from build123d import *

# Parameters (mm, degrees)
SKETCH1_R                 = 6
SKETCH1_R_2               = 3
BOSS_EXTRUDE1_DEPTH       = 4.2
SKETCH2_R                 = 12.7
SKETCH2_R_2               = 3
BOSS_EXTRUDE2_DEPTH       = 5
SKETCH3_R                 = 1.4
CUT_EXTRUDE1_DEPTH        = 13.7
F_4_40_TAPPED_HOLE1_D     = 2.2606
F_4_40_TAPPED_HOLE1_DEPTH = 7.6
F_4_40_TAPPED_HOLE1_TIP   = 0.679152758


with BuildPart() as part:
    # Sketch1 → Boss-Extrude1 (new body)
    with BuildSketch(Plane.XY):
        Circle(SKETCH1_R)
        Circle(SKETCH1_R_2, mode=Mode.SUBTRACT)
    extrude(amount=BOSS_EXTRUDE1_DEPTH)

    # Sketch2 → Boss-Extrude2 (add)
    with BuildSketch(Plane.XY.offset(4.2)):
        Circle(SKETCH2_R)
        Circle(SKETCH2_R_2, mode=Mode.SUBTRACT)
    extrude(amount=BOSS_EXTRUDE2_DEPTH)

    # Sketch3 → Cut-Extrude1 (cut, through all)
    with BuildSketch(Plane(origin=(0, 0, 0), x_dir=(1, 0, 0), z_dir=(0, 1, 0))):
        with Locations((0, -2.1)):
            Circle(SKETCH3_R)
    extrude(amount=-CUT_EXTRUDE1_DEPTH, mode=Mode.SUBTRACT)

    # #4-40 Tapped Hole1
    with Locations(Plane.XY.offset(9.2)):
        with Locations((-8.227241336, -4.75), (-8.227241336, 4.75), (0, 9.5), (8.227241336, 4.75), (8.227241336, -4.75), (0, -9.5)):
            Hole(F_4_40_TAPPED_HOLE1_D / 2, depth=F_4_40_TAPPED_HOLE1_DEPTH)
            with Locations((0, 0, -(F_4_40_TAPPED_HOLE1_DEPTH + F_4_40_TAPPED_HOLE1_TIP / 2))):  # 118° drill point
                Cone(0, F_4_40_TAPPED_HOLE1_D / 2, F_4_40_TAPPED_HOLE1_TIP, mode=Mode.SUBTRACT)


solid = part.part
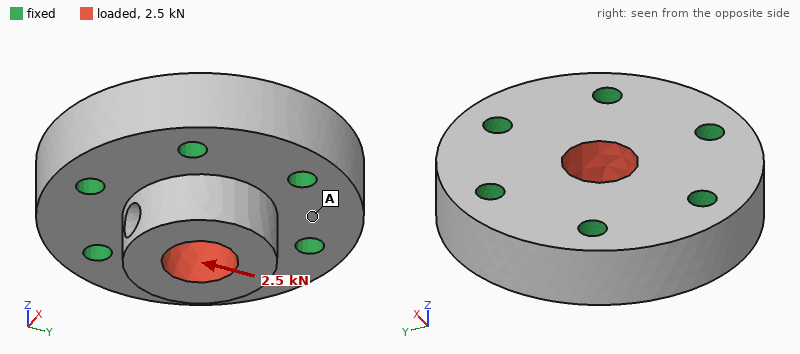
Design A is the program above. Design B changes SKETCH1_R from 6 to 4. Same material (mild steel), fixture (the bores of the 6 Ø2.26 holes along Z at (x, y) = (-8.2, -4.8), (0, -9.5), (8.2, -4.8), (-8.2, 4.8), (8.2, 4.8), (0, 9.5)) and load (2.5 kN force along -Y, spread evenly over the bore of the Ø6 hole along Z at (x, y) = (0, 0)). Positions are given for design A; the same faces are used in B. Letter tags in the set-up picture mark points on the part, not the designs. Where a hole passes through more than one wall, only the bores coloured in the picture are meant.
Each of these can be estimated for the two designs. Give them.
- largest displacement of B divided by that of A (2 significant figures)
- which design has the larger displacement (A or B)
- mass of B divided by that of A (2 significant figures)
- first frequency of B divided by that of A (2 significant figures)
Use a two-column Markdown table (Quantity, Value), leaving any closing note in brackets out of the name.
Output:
| Quantity | Value |
|---|---|
| largest displacement of B divided by that of A | 3.3 |
| which design has the larger displacement | B |
| mass of B divided by that of A | 0.90 |
| first frequency of B divided by that of A | 0.98 |
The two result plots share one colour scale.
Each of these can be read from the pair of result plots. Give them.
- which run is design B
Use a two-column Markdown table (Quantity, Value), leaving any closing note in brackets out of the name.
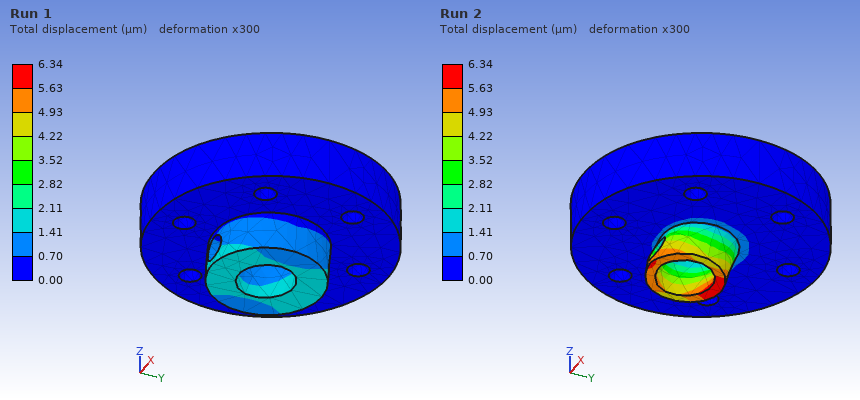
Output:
| Quantity | Value |
|---|---|
| which run is design B | Run 2 |
